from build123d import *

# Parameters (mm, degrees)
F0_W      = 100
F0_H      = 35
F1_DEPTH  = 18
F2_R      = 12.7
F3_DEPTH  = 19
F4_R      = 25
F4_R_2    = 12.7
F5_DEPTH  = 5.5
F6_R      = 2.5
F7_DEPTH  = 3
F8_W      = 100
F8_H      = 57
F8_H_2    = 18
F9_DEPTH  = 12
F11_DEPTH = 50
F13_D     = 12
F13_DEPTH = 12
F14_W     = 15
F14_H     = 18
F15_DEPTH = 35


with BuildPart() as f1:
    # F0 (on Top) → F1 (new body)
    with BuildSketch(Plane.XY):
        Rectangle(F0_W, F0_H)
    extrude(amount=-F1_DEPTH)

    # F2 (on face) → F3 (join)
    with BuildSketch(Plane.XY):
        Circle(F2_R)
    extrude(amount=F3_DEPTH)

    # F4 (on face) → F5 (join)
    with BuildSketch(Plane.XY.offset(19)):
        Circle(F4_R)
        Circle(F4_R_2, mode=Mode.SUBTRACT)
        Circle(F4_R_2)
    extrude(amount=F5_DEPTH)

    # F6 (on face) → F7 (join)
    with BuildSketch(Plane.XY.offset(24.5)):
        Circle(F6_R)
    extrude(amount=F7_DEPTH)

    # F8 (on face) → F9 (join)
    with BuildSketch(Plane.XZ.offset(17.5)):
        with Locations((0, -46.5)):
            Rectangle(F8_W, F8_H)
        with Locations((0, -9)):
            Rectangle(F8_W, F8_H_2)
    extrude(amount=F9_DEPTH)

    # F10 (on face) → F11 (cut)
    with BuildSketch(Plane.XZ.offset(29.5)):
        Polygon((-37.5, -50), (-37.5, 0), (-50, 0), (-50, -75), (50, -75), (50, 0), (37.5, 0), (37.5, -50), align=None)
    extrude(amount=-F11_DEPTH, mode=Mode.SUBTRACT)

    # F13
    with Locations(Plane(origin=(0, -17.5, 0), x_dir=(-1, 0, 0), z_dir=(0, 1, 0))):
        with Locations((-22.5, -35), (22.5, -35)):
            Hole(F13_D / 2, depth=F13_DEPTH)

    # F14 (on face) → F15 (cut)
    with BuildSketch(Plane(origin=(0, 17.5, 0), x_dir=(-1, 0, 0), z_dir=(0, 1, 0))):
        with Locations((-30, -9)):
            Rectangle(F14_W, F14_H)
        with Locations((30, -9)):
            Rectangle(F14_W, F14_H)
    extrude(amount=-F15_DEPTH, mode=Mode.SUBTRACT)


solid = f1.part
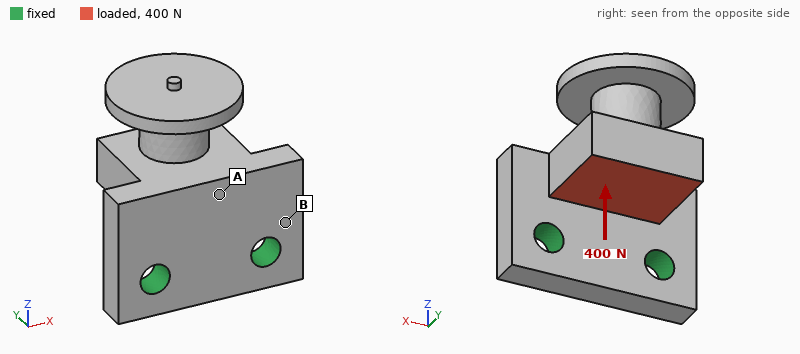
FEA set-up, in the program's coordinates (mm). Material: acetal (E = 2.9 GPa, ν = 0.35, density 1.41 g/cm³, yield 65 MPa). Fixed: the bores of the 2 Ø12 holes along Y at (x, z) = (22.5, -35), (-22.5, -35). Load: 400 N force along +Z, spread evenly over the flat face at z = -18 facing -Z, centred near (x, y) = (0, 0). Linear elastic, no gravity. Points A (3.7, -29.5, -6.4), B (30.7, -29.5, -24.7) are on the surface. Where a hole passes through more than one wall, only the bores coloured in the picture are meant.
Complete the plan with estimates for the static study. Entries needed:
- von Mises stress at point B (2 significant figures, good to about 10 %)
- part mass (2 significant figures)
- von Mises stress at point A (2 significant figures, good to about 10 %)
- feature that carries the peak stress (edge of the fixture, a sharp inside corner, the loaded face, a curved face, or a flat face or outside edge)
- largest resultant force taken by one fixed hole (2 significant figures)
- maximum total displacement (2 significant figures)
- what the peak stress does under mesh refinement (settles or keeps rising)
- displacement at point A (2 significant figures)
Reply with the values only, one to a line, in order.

4.1 MPa
130 g
1.2 MPa
edge of the fixture
210 N
0.50 mm
keeps rising
0.11 mm
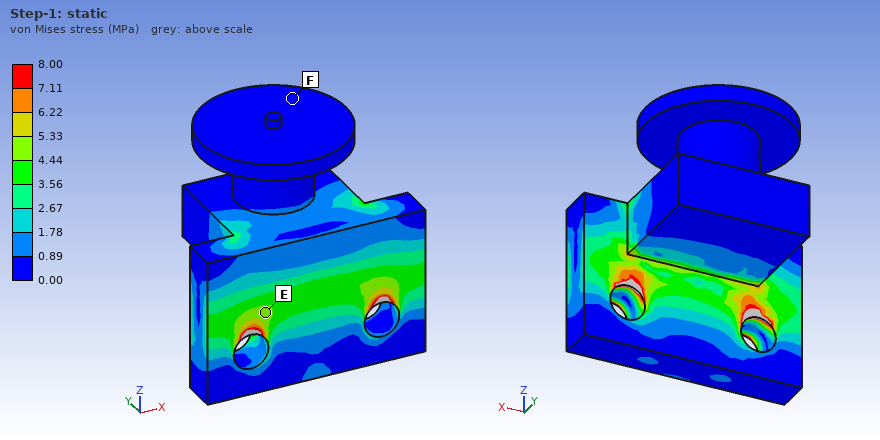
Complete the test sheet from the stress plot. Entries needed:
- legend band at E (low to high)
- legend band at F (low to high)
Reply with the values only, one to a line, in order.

4.44 to 5.33 MPa
0.00 to 0.89 MPa
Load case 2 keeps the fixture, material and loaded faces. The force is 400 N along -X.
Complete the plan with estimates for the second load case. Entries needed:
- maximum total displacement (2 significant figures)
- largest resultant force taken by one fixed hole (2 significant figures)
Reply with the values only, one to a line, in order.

0.11 mm
300 N
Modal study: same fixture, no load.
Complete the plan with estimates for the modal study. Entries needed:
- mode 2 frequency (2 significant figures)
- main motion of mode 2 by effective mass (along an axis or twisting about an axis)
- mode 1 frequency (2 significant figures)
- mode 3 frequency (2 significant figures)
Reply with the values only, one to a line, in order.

1400 Hz
along X
550 Hz
1800 Hz
